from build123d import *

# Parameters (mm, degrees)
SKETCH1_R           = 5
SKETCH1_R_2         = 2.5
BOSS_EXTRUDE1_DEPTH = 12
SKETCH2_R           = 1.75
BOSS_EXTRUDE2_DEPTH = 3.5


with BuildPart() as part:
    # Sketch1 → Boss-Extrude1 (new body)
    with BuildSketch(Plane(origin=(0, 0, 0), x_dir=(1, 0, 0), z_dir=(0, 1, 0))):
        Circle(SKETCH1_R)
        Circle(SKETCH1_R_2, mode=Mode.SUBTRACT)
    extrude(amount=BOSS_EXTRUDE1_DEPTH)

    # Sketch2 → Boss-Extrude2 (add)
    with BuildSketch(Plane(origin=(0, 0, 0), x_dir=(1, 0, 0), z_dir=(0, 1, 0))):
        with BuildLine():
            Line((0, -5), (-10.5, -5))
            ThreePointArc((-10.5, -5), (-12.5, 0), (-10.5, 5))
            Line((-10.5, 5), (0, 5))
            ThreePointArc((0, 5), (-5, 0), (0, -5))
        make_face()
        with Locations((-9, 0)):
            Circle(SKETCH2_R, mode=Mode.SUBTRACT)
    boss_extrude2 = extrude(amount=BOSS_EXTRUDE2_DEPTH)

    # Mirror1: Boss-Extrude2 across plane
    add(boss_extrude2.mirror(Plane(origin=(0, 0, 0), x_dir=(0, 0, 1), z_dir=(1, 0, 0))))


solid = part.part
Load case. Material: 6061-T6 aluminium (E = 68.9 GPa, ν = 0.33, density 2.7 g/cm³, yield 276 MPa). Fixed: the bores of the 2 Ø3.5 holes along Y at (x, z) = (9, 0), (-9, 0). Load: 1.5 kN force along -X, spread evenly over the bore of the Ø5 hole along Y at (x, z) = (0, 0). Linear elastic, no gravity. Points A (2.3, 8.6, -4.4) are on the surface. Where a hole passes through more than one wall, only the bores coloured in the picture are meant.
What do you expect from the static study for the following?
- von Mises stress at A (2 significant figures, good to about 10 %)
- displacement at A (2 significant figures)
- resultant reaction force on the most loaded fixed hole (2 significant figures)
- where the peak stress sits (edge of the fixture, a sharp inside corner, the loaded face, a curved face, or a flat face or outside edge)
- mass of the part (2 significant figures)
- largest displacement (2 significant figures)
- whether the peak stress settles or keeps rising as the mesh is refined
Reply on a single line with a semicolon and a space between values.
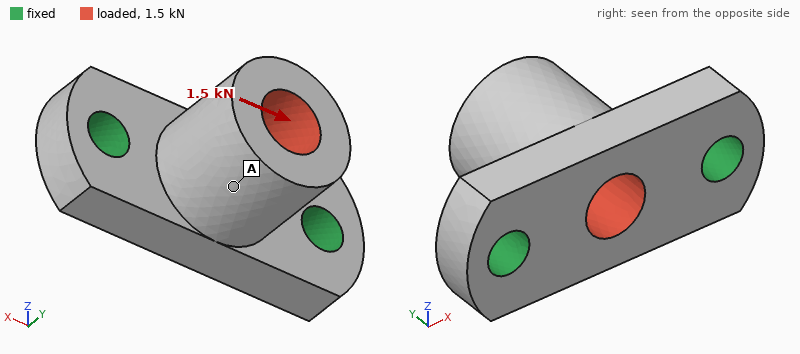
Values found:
16 MPa; 12 µm; 890 N; edge of the fixture; 3.2 g; 18 µm; keeps rising
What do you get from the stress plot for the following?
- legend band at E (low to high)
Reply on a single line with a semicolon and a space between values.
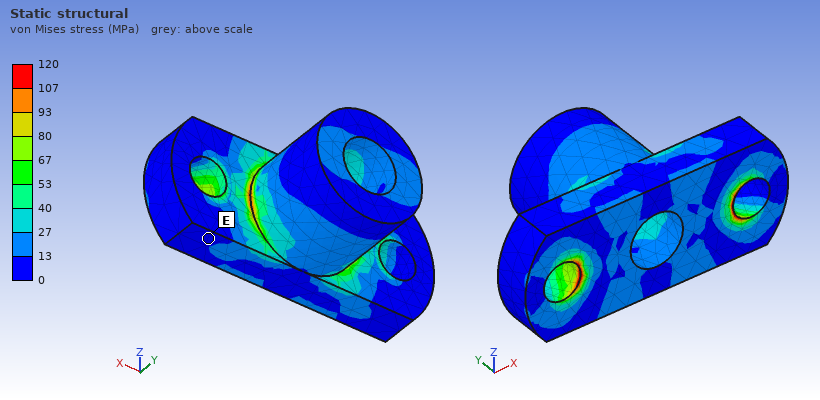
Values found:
0 to 13 MPa
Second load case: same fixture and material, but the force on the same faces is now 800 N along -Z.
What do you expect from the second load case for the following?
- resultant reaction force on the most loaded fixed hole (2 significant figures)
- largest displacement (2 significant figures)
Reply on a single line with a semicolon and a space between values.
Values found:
400 N; 35 µm
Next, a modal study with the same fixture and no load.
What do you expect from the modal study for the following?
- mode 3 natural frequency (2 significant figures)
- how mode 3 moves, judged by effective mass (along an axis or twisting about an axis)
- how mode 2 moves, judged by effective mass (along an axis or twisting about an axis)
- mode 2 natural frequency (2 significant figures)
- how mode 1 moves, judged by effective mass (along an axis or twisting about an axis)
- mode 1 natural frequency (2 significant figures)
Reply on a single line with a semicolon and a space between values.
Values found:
42 kHz; along Y; along X; 39 kHz; along Z; 20 kHz
